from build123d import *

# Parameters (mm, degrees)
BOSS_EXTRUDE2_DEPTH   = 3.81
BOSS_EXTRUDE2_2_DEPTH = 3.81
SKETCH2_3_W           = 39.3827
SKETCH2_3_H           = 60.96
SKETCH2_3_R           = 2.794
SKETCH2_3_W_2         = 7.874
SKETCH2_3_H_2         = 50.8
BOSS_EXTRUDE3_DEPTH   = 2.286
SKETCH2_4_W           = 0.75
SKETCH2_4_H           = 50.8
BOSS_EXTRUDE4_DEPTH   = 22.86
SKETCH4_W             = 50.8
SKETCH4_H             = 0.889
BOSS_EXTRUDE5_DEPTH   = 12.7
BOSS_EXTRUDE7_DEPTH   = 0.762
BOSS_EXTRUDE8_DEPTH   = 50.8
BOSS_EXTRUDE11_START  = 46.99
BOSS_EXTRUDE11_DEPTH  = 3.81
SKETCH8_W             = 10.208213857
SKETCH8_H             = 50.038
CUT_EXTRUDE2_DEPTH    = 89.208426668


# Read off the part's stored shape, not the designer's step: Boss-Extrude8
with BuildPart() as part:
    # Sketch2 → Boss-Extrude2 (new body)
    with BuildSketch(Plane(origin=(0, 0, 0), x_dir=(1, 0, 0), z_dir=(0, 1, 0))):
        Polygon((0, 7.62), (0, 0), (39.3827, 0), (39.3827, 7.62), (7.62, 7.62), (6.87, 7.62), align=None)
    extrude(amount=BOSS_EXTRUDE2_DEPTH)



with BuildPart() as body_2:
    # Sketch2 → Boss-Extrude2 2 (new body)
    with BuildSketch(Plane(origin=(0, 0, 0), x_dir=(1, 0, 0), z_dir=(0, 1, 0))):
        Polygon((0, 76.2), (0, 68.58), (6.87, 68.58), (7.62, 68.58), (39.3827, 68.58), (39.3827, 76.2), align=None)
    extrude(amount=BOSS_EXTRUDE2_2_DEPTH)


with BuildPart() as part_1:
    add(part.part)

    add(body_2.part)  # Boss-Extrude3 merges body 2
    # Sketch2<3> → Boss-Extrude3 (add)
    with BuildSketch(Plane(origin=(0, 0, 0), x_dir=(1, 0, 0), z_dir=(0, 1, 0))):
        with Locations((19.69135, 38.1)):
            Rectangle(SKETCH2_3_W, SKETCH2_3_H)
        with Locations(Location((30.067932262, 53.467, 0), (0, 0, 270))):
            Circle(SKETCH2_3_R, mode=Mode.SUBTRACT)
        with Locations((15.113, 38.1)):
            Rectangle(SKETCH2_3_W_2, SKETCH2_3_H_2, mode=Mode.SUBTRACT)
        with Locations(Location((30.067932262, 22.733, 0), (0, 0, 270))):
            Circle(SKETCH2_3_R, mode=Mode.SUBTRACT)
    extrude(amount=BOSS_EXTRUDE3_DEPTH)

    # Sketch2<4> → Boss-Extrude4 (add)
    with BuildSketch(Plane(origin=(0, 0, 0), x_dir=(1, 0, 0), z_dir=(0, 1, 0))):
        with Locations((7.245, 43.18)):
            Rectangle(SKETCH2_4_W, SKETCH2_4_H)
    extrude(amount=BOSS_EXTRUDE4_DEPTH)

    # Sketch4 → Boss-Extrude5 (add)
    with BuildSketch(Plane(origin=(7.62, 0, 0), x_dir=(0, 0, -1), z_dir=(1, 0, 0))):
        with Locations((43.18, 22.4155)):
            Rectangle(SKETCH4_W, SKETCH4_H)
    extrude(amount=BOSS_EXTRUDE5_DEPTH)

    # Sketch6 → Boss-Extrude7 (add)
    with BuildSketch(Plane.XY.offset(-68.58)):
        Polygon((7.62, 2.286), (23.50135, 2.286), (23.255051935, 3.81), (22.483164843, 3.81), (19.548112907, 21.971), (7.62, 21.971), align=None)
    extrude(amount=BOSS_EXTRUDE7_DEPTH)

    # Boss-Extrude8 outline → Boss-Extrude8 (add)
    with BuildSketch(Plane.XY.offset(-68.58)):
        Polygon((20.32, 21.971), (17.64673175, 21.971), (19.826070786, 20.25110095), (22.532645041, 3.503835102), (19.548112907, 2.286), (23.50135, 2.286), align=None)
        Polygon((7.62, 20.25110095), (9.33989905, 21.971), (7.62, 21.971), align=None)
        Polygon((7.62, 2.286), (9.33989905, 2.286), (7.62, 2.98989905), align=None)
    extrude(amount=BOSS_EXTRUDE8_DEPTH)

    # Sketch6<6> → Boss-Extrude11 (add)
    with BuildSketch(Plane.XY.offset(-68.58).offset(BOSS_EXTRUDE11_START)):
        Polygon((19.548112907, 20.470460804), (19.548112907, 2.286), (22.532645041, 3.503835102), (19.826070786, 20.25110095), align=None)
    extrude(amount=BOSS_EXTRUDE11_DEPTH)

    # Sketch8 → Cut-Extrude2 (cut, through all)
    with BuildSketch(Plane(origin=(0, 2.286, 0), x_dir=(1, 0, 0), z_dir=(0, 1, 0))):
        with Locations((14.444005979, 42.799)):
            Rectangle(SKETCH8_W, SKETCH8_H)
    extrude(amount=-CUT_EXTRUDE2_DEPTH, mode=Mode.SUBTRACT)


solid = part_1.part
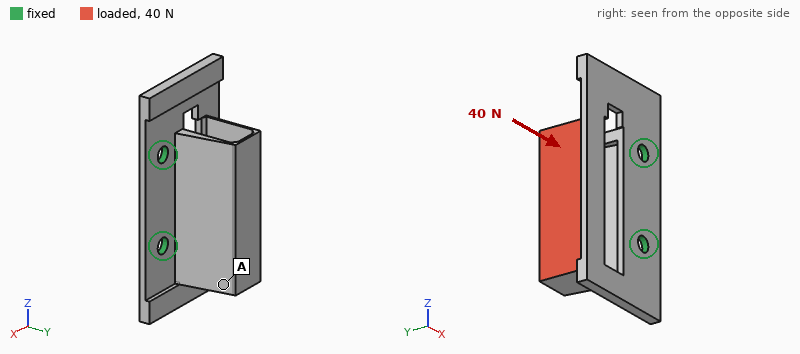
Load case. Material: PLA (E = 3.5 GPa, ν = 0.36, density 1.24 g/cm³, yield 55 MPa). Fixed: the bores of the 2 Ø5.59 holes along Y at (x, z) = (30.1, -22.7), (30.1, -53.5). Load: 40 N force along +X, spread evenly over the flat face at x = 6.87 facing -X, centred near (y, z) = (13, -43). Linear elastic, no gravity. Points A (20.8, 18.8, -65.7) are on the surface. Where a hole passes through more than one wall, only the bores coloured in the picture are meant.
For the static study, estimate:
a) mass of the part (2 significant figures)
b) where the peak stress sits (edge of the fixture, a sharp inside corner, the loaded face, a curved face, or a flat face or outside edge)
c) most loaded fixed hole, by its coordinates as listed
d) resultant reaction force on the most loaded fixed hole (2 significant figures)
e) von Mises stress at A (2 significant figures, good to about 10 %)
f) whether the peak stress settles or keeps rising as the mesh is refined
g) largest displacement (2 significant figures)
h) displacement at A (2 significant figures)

11 g
a sharp inside corner
(30.1, -53.5)
25 N
1.3 MPa
keeps rising
0.86 mm
0.53 mm
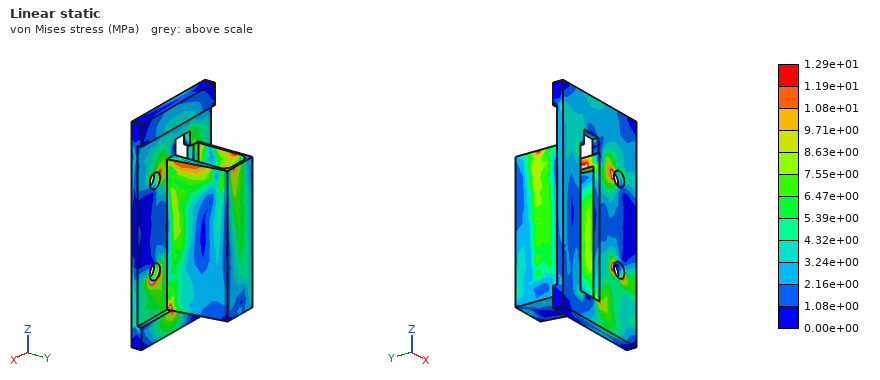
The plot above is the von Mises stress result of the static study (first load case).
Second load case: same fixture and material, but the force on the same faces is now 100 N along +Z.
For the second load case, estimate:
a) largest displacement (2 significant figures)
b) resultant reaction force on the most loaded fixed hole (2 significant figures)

0.41 mm
84 N
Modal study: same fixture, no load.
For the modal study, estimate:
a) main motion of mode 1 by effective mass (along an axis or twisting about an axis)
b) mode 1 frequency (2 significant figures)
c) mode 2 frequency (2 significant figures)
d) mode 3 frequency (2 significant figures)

along Y
420 Hz
880 Hz
1200 Hz
